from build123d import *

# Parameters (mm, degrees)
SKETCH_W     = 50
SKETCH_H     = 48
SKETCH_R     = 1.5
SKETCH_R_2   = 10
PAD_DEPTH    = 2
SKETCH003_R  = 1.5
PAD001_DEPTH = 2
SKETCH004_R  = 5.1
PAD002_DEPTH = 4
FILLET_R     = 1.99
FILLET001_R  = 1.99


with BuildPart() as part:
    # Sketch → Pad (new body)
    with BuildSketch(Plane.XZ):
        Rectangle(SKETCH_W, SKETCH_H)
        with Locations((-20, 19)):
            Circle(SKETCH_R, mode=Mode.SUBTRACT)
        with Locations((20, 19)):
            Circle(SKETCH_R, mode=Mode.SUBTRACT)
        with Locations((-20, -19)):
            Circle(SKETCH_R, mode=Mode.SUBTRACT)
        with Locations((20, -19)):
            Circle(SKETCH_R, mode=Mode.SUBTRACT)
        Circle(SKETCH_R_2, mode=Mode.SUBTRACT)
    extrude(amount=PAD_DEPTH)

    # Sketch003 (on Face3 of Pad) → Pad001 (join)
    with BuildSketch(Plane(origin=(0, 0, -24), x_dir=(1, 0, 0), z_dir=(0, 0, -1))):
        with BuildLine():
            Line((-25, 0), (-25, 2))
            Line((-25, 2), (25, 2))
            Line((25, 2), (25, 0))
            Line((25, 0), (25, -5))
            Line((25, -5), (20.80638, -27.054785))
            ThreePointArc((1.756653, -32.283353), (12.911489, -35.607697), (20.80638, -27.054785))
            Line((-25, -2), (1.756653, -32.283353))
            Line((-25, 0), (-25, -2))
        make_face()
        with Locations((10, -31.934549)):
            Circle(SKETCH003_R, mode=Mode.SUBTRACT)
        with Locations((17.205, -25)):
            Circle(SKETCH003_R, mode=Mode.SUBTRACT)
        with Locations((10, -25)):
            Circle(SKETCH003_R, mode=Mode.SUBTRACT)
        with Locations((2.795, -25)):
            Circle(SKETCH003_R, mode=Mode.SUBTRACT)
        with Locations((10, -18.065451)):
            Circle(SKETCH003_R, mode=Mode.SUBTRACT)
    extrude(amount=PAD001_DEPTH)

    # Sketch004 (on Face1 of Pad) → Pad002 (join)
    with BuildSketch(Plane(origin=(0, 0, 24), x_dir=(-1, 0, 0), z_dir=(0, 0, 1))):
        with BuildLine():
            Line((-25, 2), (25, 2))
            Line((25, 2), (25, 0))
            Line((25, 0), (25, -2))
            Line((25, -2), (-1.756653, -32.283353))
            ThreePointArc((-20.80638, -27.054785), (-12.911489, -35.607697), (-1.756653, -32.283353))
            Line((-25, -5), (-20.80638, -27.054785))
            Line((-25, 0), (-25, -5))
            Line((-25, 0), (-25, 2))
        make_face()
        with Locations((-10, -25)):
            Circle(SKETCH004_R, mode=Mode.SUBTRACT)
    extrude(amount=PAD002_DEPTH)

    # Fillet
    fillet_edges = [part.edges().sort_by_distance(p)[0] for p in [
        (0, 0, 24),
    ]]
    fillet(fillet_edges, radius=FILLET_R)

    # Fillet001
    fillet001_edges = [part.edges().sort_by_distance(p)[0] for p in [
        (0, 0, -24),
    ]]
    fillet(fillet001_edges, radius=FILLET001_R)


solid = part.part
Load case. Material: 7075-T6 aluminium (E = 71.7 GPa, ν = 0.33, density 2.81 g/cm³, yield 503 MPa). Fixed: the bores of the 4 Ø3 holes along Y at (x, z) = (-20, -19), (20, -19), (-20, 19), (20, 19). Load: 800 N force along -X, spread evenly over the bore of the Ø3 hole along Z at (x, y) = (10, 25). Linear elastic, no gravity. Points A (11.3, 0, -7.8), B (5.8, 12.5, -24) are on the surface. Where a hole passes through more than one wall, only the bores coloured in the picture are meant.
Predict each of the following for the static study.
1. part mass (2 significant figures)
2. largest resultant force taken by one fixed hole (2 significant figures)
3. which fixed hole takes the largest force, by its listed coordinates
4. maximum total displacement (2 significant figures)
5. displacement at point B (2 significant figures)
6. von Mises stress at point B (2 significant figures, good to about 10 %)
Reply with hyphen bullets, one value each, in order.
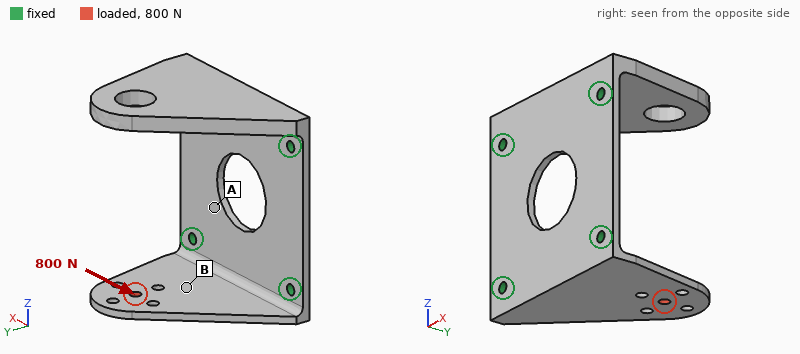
- 32 g
- 700 N
- (-20, -19)
- 0.15 mm
- 0.042 mm
- 32 MPa
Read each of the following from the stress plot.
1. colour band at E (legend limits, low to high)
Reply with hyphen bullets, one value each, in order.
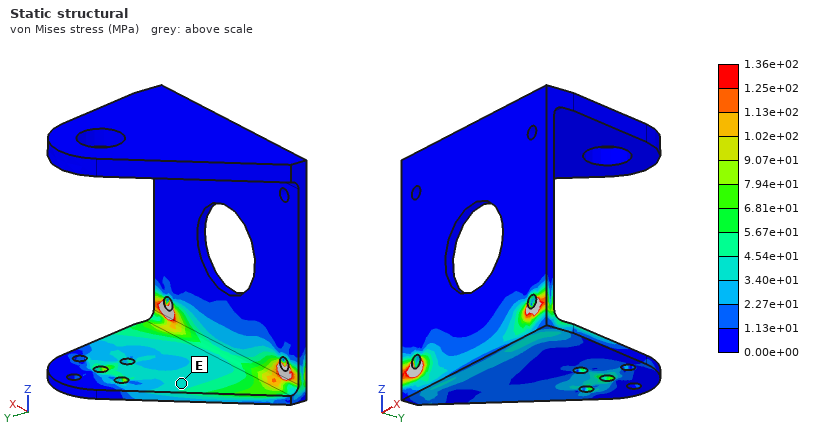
- 3.40e+01 to 4.54e+01 MPa
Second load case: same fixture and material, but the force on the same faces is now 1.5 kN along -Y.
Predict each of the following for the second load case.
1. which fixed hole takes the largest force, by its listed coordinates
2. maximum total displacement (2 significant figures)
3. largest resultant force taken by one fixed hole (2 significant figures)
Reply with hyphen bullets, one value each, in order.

- (20, -19)
- 0.55 mm
- 1.2 kN
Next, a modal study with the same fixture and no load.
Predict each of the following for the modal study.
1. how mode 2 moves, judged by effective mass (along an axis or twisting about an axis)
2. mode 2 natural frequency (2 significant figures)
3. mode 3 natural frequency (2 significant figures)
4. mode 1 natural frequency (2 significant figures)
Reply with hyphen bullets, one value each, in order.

- along Z
- 1500 Hz
- 4600 Hz
- 1400 Hz
